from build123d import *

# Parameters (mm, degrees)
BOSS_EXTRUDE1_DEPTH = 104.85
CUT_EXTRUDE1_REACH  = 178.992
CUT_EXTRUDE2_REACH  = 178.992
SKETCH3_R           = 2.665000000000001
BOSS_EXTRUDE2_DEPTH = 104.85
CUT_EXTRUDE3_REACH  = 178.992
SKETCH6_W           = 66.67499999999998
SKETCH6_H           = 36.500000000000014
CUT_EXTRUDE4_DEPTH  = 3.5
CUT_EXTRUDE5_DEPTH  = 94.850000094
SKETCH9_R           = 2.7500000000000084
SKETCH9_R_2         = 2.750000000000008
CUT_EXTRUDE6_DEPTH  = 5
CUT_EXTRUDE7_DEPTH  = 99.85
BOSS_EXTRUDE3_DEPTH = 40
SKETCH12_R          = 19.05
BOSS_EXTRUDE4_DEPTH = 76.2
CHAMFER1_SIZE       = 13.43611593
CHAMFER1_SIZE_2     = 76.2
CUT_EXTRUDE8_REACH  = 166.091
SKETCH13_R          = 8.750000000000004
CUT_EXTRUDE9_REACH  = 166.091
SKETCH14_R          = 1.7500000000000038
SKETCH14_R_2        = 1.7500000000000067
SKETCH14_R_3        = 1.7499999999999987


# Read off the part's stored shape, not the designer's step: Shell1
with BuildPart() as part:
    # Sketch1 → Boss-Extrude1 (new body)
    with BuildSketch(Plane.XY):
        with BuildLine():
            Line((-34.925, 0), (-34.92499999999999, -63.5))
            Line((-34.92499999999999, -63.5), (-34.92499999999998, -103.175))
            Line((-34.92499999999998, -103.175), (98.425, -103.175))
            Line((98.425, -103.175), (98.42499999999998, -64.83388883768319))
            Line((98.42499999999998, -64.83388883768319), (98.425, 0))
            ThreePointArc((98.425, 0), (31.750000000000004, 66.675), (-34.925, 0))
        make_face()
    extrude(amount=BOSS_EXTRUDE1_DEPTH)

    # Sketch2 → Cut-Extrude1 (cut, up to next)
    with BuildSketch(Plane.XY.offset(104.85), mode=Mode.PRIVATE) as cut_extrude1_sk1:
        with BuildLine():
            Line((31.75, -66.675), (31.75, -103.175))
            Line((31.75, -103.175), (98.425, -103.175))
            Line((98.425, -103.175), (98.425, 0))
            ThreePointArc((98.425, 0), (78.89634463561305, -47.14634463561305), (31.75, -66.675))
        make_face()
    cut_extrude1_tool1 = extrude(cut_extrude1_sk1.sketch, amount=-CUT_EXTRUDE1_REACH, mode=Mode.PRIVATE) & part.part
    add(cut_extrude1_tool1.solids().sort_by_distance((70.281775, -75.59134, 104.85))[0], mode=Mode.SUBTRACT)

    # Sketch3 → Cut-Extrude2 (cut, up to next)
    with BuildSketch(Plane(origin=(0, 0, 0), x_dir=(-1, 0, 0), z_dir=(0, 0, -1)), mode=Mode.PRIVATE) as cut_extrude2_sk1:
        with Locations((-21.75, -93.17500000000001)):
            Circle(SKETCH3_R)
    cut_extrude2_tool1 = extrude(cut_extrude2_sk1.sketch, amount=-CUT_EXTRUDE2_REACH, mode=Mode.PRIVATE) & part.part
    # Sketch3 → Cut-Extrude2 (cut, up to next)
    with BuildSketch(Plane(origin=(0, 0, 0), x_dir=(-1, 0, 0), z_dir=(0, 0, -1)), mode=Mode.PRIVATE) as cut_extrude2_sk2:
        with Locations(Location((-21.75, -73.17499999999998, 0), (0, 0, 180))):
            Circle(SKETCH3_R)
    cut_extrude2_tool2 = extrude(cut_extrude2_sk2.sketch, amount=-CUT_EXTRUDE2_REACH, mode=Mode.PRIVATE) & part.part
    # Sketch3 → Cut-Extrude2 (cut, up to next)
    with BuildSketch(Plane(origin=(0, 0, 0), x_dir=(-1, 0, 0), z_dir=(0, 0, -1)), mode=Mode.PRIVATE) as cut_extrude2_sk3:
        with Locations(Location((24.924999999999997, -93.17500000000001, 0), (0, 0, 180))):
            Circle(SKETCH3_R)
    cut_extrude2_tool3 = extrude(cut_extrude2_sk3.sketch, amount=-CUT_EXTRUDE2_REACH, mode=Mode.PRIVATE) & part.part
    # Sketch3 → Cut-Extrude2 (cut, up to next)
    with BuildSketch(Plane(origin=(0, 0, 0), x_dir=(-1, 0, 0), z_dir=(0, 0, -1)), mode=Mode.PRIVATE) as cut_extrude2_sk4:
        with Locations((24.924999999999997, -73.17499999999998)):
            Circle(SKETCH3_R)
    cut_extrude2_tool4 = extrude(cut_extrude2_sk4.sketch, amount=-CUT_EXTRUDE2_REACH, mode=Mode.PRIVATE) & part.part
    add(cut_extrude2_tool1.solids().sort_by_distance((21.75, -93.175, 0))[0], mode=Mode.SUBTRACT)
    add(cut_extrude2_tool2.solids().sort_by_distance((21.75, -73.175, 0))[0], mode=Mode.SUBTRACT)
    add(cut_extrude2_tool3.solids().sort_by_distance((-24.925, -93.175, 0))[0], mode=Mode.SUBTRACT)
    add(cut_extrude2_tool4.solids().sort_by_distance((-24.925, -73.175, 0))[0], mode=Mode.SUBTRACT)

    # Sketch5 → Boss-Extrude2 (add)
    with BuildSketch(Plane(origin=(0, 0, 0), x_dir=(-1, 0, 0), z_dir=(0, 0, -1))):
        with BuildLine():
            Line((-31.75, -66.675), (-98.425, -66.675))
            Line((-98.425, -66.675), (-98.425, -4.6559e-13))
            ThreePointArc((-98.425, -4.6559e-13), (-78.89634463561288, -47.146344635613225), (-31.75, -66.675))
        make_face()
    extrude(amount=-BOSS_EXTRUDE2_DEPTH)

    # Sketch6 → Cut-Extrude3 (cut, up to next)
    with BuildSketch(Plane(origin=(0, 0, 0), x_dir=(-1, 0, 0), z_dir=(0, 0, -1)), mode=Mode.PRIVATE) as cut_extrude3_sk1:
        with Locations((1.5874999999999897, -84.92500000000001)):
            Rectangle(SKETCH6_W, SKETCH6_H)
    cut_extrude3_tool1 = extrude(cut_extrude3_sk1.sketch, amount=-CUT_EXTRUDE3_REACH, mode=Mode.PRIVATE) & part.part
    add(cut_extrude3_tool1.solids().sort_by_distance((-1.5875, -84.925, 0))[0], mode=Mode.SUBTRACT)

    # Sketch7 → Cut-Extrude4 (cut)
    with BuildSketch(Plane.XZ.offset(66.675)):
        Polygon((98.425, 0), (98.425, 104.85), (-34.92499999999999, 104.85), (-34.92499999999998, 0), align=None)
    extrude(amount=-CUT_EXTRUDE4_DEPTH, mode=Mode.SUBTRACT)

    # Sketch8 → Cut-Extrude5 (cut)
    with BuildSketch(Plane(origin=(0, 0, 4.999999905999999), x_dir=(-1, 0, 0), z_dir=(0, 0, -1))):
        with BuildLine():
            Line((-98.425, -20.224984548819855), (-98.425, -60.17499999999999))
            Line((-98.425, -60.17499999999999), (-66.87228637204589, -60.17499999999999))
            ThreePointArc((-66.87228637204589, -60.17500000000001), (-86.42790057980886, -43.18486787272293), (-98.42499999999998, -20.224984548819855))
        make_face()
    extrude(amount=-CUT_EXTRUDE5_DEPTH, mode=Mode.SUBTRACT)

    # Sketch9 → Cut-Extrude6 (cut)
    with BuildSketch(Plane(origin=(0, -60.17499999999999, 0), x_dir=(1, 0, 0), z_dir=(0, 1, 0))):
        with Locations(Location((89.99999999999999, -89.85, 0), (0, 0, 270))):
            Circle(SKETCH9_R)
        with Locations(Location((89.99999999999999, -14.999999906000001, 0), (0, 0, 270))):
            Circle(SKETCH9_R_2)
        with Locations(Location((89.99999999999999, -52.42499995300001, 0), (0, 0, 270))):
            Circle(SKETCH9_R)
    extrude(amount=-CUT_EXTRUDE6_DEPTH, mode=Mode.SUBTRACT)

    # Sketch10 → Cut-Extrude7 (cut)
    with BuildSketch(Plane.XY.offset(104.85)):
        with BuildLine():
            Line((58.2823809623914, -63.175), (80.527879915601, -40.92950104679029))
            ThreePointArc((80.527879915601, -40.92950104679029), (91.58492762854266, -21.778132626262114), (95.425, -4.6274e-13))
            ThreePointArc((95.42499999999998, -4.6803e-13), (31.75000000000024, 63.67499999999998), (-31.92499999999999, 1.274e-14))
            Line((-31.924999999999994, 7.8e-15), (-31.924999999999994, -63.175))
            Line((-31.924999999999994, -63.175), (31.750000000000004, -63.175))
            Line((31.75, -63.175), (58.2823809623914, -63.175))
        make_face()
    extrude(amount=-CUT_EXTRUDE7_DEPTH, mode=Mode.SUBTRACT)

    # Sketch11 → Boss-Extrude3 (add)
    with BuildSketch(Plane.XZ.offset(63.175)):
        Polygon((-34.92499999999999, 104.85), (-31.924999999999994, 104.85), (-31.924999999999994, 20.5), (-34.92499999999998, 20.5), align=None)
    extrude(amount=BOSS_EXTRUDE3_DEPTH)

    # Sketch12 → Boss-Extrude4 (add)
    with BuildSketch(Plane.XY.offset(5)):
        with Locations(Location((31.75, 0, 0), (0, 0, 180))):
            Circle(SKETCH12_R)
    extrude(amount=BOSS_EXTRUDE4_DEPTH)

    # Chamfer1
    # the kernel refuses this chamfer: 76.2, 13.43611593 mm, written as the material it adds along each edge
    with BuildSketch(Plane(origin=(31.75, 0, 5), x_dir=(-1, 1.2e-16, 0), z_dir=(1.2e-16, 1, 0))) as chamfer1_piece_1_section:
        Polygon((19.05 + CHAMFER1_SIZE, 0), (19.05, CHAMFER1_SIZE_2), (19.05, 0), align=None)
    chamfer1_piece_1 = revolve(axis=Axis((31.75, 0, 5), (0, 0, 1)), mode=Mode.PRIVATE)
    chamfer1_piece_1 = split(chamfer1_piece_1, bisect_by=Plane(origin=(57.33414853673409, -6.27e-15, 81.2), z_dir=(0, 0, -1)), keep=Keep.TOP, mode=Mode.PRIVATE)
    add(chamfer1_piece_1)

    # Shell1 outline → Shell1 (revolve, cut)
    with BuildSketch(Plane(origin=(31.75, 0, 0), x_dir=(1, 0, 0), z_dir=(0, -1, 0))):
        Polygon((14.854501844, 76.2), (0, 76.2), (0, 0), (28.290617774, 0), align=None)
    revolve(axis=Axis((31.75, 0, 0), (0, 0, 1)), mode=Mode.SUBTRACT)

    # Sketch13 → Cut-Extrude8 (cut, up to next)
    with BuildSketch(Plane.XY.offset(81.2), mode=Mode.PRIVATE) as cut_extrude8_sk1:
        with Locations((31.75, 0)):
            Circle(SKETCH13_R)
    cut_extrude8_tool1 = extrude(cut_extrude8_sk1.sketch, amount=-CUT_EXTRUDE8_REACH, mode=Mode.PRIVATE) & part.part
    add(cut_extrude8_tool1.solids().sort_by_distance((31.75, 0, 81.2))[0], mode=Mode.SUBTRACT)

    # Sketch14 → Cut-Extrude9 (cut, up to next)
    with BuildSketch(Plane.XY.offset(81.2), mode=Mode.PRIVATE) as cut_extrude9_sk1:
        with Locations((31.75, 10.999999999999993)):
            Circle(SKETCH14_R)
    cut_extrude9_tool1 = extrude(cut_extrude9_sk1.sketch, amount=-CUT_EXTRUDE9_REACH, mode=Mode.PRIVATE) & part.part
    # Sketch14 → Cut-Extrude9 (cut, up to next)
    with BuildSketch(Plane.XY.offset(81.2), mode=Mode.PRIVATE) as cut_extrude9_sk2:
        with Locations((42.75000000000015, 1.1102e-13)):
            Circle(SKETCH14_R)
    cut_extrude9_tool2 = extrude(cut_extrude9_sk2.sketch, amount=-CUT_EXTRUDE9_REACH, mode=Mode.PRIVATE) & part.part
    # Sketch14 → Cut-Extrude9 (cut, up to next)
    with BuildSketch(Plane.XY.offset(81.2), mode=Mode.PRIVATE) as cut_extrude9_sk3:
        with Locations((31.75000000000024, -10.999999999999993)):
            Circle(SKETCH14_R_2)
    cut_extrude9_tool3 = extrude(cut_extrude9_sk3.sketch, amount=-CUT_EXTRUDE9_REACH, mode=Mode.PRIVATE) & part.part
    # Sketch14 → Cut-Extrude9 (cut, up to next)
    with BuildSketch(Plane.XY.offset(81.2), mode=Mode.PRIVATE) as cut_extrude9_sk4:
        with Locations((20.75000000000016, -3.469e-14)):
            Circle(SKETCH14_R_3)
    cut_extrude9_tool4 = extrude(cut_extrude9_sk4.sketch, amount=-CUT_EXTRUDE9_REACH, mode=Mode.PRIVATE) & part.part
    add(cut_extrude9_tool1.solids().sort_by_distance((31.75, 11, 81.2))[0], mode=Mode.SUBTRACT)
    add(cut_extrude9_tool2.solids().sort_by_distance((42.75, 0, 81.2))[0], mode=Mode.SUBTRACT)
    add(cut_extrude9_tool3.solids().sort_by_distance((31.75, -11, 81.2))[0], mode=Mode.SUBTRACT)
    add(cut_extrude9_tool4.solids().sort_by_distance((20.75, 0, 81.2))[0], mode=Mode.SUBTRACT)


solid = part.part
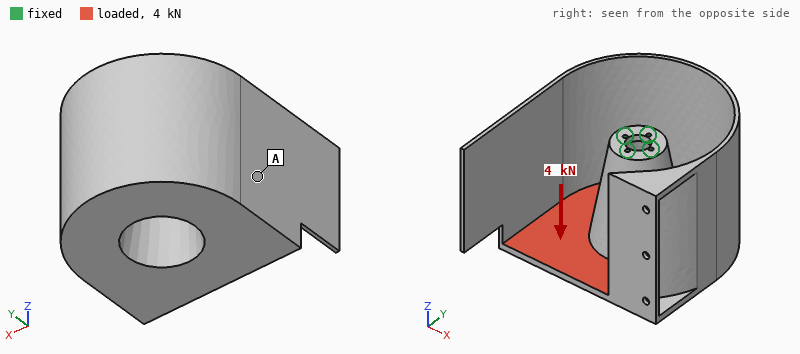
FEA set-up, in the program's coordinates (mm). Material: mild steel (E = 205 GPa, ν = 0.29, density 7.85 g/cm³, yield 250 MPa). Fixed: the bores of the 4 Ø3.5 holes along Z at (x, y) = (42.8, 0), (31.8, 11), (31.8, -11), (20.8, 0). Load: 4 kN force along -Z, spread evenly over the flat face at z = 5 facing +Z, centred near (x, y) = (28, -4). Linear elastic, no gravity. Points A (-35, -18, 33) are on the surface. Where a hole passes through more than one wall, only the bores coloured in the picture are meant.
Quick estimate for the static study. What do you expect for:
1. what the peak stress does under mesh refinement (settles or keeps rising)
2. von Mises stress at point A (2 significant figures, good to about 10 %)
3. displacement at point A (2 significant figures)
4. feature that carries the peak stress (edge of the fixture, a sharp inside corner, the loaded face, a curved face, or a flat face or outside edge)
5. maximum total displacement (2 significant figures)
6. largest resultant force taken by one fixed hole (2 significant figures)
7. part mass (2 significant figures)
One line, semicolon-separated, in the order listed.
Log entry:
keeps rising; 8.2 MPa; 0.078 mm; edge of the fixture; 0.17 mm; 1.6 kN; 2.1 kg
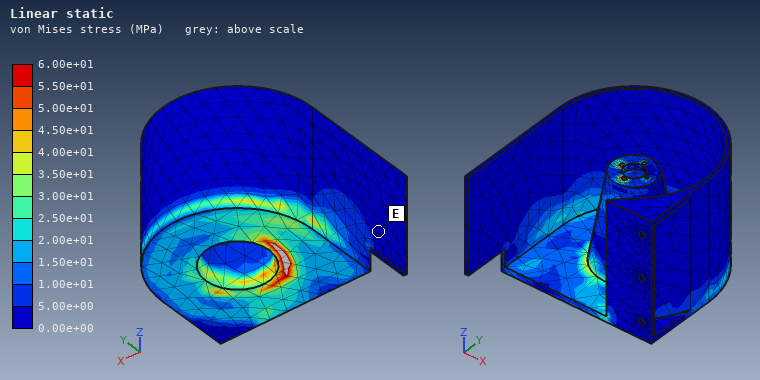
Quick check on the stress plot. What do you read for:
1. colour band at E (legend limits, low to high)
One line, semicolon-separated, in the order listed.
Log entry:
0.00e+00 to 5.00e+00 MPa
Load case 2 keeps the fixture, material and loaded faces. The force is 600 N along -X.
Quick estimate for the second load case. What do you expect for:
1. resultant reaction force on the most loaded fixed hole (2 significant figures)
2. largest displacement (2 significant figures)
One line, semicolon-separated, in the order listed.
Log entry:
1.4 kN; 29 µm
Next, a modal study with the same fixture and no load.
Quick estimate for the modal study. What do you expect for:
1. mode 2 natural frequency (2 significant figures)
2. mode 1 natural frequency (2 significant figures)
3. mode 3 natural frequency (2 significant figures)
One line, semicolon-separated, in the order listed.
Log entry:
350 Hz; 240 Hz; 420 Hz
